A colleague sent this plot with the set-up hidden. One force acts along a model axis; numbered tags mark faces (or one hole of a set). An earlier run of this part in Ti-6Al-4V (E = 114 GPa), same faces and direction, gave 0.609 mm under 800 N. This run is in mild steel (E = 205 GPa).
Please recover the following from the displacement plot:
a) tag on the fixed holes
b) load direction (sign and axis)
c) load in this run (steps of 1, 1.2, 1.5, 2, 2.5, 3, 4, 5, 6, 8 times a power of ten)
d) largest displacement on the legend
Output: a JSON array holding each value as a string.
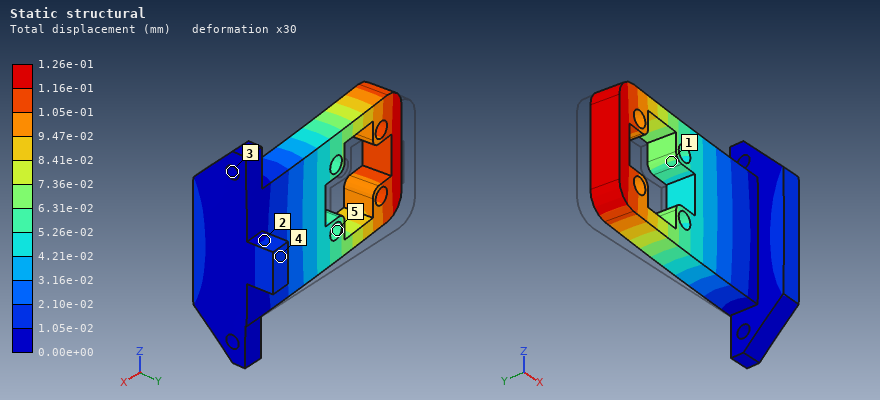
["3", "-Y", "300 N", "1.26e-01 mm"]
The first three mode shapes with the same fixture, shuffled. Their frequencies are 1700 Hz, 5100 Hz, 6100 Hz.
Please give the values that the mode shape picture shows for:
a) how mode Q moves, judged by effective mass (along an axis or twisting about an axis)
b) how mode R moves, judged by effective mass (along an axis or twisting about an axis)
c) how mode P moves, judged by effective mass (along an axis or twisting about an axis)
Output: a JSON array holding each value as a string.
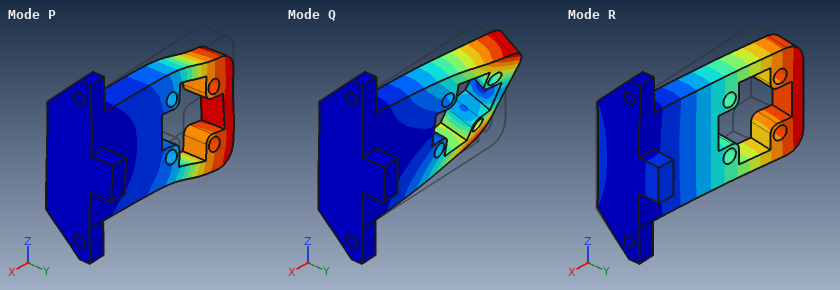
["twisting about X", "along Y", "along Z"]
